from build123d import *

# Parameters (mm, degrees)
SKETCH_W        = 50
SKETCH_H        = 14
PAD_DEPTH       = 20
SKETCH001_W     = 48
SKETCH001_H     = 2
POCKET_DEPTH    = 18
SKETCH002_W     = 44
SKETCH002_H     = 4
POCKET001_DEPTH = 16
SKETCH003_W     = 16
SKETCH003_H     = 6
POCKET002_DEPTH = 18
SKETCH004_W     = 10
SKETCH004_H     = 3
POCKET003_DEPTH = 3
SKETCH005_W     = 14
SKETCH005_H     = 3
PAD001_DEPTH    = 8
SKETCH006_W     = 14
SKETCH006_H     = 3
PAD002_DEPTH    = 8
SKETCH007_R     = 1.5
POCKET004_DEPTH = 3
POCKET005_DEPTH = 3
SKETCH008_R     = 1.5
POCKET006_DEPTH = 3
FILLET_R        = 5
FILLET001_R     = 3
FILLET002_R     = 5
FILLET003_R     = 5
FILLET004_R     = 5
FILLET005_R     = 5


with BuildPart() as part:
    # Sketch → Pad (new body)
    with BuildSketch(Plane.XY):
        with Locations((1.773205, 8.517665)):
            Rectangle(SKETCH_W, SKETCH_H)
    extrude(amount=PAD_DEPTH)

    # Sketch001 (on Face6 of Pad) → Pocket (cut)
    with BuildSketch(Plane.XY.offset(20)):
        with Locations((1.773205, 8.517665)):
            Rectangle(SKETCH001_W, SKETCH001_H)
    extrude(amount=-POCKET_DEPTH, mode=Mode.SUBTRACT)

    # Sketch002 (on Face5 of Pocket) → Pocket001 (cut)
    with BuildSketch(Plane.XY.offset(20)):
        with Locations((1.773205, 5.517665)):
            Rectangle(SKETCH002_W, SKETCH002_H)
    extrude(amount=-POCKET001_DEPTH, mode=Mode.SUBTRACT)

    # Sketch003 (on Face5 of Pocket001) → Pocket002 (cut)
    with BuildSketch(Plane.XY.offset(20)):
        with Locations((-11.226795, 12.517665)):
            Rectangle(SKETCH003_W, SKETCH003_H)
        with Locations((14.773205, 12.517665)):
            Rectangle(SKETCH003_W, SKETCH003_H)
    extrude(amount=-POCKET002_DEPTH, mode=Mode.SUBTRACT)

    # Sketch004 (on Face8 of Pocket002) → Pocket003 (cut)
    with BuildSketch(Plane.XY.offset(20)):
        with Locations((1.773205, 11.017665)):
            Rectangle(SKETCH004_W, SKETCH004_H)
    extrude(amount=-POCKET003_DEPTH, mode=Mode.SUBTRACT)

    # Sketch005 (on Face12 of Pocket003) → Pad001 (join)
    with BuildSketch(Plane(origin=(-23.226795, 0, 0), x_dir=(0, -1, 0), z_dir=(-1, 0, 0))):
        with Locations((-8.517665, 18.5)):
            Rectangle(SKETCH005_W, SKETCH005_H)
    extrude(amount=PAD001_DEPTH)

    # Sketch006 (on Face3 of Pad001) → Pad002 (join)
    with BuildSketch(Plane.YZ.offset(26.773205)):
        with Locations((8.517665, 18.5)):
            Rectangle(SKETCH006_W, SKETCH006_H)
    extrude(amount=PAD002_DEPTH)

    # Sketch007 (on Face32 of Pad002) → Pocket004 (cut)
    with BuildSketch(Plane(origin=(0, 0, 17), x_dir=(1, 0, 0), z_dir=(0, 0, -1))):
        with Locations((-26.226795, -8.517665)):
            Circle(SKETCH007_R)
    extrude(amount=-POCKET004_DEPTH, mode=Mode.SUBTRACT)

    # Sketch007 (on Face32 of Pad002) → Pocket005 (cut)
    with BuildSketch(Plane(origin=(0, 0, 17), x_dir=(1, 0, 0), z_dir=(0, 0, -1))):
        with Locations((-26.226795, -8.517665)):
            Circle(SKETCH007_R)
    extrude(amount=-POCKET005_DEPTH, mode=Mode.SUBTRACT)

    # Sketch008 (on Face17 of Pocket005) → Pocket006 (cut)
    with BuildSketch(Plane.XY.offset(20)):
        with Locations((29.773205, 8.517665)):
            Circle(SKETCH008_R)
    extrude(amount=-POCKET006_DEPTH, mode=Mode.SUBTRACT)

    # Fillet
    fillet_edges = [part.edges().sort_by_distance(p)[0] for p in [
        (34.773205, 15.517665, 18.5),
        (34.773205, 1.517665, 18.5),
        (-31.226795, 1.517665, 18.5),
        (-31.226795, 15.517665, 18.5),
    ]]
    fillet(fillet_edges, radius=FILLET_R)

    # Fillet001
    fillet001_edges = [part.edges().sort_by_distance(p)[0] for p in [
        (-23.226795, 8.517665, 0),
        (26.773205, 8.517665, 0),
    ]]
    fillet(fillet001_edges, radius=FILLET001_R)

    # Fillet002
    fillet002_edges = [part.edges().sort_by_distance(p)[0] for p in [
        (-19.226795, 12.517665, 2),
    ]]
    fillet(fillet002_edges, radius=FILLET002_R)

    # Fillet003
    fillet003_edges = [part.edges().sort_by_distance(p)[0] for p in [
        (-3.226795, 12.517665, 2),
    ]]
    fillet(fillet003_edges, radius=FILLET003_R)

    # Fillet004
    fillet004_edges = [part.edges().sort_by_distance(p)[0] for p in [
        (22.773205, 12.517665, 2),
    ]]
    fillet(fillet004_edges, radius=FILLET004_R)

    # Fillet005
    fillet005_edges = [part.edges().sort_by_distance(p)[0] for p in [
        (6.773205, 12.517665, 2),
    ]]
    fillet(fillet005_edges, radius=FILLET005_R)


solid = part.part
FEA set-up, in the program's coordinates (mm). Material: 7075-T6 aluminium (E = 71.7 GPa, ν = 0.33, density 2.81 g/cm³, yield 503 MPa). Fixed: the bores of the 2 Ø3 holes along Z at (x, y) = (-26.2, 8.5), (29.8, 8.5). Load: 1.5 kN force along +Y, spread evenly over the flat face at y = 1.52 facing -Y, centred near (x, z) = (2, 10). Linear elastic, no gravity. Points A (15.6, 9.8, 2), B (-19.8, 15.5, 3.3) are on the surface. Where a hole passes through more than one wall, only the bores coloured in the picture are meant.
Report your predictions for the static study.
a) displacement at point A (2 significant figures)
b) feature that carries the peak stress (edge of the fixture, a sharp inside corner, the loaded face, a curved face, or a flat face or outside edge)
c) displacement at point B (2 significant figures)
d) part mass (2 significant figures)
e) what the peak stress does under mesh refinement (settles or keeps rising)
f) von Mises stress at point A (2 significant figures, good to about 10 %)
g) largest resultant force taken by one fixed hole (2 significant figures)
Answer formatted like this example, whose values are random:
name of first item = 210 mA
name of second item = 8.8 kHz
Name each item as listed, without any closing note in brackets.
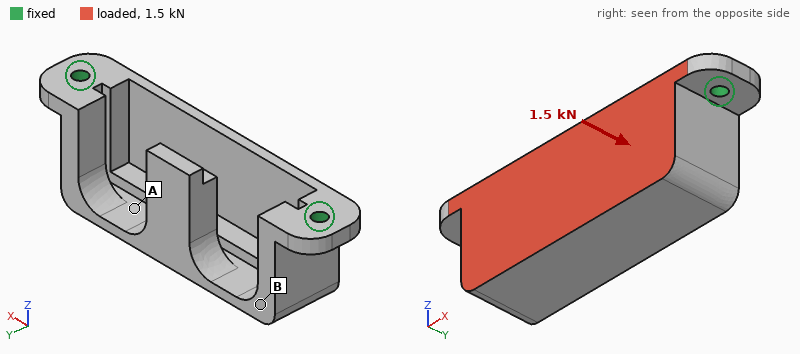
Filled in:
displacement at point A = 0.15 mm
feature that carries the peak stress = edge of the fixture
displacement at point B = 0.13 mm
part mass = 18 g
what the peak stress does under mesh refinement = keeps rising
von Mises stress at point A = 63 MPa
largest resultant force taken by one fixed hole = 830 N
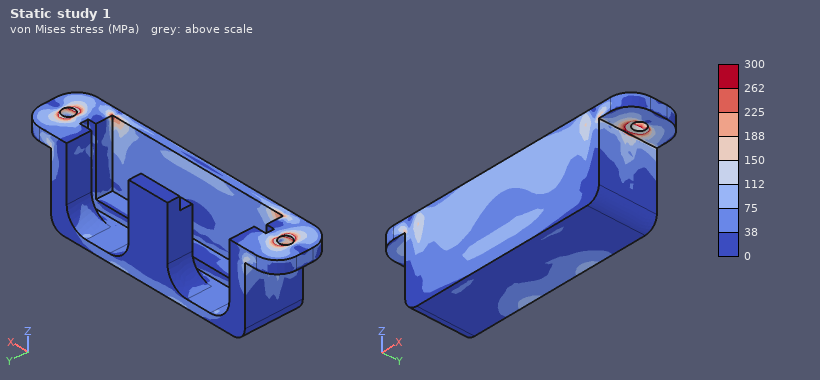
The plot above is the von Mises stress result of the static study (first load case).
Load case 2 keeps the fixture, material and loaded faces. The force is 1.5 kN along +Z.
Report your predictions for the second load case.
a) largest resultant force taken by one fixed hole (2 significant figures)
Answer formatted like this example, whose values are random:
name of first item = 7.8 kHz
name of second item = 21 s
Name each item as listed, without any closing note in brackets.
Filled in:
largest resultant force taken by one fixed hole = 830 N
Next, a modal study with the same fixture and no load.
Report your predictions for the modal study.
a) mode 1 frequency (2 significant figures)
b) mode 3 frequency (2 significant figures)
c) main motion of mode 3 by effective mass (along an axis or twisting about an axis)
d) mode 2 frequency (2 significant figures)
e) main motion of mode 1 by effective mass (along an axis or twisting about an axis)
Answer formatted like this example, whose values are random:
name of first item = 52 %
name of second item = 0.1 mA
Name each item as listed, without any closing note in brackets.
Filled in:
mode 1 frequency = 3600 Hz
mode 3 frequency = 5200 Hz
main motion of mode 3 by effective mass = along X
mode 2 frequency = 4300 Hz
main motion of mode 1 by effective mass = along Y
